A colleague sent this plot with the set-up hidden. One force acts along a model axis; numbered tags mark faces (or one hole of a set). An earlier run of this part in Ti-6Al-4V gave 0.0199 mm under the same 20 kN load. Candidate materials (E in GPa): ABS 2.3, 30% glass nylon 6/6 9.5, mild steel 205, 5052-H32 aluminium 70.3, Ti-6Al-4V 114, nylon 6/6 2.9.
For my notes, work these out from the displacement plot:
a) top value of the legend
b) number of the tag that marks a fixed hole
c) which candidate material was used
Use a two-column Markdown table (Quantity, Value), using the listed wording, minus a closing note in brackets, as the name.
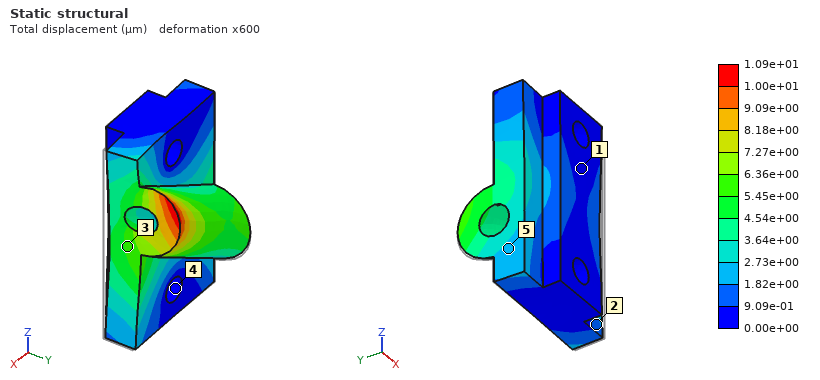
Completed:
| Quantity | Value |
|---|---|
| top value of the legend | 1.09e+01 µm |
| number of the tag that marks a fixed hole | 4 |
| which candidate material was used | mild steel |
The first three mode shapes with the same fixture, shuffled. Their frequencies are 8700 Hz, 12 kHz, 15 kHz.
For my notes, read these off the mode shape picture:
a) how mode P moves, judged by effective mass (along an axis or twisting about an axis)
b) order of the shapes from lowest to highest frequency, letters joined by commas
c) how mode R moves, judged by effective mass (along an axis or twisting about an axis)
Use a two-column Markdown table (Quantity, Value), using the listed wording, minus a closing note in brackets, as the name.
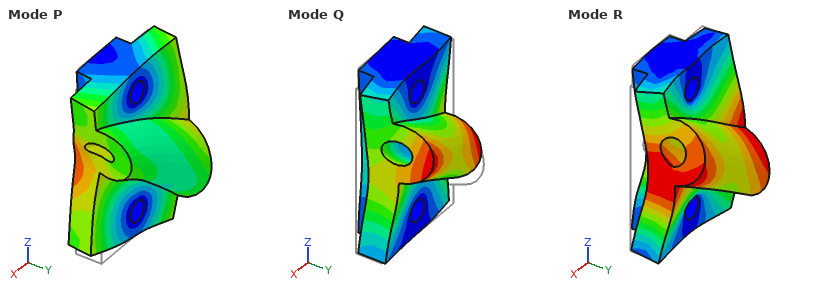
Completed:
| Quantity | Value |
|---|---|
| how mode P moves, judged by effective mass | along X |
| order of the shapes from lowest to highest frequency, letters joined by commas | Q, R, P |
| how mode R moves, judged by effective mass | along Y |
